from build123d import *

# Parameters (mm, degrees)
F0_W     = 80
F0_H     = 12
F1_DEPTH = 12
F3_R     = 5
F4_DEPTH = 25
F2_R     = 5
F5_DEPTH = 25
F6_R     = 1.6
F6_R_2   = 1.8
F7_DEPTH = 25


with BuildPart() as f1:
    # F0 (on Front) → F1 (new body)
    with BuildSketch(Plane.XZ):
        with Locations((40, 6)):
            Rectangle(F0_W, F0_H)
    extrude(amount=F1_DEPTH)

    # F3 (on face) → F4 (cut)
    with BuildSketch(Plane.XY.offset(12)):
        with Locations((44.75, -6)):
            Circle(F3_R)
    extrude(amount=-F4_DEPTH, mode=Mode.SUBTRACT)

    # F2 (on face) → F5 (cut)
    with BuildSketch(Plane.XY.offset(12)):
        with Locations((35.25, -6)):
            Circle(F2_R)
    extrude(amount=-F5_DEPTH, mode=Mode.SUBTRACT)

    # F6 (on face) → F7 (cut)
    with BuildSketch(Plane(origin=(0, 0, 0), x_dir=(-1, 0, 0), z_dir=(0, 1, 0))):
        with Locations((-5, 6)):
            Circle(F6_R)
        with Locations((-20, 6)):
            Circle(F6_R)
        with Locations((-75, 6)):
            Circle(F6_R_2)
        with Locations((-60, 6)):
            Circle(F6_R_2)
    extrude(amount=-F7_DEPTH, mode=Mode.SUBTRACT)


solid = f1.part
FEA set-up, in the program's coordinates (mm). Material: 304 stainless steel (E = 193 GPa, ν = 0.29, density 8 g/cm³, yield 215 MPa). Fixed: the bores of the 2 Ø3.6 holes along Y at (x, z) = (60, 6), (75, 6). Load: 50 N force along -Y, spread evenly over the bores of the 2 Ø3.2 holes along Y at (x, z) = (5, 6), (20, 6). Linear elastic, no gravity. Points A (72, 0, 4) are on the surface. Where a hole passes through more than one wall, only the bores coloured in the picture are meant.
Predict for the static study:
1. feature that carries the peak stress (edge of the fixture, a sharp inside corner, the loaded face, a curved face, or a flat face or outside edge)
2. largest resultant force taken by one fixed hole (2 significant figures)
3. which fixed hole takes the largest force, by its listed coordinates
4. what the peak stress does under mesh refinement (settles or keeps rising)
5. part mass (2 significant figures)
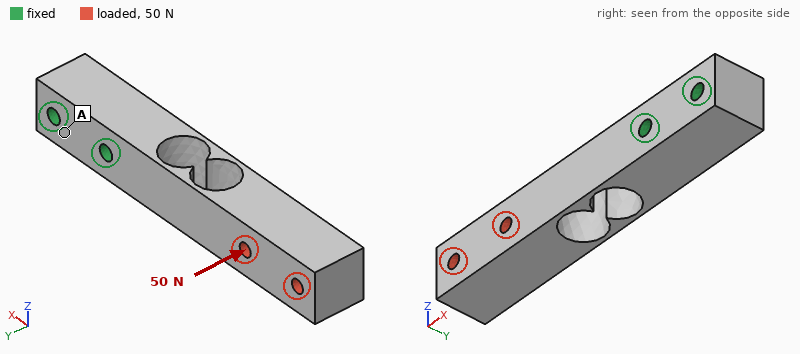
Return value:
a sharp inside corner
72 N
(60, 6)
keeps rising
74 g
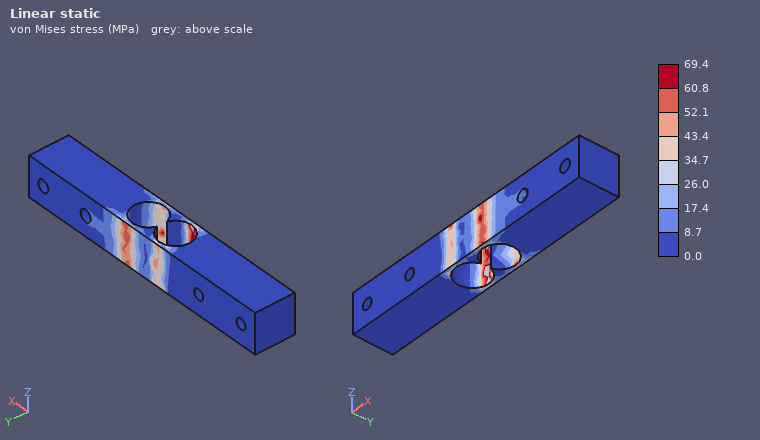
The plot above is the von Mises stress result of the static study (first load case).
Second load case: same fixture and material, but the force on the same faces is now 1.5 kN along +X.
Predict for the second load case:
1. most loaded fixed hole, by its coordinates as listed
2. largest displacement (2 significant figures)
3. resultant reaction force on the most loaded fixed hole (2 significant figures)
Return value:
(60, 6)
7.9 µm
1.4 kN
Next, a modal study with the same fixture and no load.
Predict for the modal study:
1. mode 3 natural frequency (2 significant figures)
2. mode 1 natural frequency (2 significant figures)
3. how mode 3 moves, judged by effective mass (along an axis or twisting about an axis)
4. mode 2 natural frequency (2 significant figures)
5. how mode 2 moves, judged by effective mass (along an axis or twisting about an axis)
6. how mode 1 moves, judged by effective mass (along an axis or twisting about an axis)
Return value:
5900 Hz
1100 Hz
twisting about X
1500 Hz
along Z
along Y
